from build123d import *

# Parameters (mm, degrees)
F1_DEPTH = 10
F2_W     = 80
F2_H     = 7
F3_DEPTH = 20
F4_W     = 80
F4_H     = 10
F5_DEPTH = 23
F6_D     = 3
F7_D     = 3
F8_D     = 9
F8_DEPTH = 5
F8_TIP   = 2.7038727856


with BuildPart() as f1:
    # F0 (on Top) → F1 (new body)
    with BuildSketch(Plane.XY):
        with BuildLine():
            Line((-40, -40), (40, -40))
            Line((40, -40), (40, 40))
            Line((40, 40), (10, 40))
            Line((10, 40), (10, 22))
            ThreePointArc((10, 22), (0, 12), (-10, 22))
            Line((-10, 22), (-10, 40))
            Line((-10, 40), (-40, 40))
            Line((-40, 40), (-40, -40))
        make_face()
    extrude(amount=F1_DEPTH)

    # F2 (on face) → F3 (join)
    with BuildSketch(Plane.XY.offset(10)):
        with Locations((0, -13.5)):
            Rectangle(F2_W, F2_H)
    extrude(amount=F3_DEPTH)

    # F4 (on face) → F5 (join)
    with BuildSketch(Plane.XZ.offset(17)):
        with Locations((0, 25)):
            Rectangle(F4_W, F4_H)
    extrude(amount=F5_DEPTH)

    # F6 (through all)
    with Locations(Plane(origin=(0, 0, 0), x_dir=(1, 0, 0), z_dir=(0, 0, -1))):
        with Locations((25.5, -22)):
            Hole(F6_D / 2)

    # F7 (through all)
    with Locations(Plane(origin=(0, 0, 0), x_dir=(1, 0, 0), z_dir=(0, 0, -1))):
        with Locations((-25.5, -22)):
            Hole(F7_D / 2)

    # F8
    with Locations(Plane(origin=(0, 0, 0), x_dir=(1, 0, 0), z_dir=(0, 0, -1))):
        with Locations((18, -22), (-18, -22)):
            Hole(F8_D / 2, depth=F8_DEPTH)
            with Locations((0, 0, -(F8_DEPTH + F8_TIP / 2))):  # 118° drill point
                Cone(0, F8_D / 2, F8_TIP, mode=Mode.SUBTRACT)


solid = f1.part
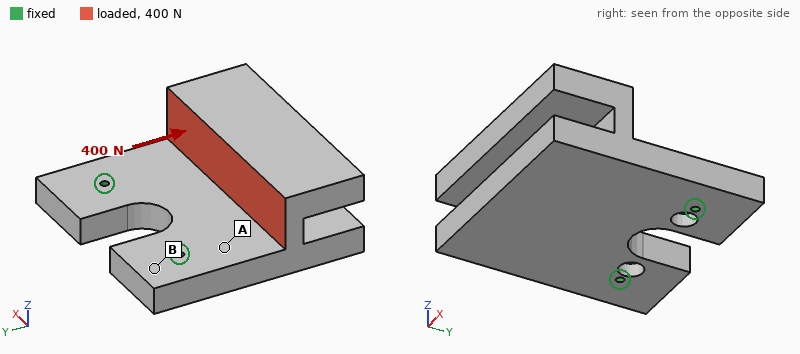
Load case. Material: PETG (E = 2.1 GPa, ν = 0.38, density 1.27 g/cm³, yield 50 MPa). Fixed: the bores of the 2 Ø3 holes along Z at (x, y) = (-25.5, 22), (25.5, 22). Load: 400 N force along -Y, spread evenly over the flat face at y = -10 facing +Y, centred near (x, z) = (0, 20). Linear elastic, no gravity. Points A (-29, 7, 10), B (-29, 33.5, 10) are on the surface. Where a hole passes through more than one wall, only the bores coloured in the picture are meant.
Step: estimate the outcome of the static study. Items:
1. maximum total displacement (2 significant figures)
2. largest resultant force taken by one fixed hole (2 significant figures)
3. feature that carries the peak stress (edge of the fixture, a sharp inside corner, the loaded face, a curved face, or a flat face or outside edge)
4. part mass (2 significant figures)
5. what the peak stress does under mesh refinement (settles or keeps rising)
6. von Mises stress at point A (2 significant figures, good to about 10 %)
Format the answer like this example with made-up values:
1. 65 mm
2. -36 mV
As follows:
1. 1.3 mm
2. 200 N
3. edge of the fixture
4. 110 g
5. keeps rising
6. 5.6 MPa
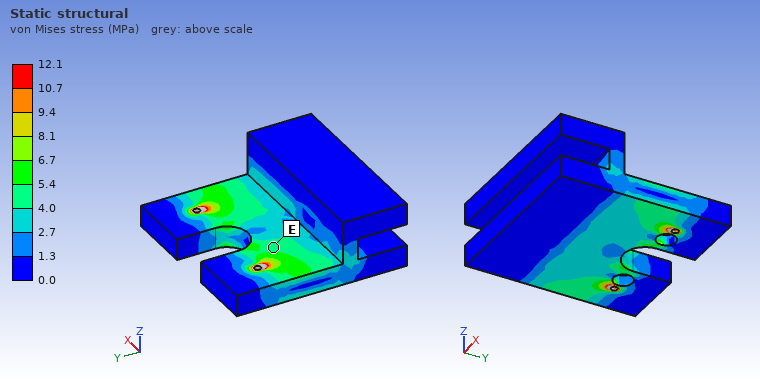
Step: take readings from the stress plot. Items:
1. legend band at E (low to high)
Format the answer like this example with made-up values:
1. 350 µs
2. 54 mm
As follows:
1. 4.0 to 5.4 MPa
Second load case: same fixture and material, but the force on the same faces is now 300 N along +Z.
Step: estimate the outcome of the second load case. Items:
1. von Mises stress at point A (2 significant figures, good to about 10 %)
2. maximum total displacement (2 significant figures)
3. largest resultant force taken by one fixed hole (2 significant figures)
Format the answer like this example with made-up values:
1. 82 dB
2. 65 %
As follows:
1. 4.4 MPa
2. 1.1 mm
3. 150 N
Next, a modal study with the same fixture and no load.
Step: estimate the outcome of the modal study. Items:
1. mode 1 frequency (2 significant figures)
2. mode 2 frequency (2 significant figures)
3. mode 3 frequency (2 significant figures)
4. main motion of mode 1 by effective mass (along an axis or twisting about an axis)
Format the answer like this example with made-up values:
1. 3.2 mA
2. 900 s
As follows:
1. 270 Hz
2. 670 Hz
3. 1100 Hz
4. along Z
